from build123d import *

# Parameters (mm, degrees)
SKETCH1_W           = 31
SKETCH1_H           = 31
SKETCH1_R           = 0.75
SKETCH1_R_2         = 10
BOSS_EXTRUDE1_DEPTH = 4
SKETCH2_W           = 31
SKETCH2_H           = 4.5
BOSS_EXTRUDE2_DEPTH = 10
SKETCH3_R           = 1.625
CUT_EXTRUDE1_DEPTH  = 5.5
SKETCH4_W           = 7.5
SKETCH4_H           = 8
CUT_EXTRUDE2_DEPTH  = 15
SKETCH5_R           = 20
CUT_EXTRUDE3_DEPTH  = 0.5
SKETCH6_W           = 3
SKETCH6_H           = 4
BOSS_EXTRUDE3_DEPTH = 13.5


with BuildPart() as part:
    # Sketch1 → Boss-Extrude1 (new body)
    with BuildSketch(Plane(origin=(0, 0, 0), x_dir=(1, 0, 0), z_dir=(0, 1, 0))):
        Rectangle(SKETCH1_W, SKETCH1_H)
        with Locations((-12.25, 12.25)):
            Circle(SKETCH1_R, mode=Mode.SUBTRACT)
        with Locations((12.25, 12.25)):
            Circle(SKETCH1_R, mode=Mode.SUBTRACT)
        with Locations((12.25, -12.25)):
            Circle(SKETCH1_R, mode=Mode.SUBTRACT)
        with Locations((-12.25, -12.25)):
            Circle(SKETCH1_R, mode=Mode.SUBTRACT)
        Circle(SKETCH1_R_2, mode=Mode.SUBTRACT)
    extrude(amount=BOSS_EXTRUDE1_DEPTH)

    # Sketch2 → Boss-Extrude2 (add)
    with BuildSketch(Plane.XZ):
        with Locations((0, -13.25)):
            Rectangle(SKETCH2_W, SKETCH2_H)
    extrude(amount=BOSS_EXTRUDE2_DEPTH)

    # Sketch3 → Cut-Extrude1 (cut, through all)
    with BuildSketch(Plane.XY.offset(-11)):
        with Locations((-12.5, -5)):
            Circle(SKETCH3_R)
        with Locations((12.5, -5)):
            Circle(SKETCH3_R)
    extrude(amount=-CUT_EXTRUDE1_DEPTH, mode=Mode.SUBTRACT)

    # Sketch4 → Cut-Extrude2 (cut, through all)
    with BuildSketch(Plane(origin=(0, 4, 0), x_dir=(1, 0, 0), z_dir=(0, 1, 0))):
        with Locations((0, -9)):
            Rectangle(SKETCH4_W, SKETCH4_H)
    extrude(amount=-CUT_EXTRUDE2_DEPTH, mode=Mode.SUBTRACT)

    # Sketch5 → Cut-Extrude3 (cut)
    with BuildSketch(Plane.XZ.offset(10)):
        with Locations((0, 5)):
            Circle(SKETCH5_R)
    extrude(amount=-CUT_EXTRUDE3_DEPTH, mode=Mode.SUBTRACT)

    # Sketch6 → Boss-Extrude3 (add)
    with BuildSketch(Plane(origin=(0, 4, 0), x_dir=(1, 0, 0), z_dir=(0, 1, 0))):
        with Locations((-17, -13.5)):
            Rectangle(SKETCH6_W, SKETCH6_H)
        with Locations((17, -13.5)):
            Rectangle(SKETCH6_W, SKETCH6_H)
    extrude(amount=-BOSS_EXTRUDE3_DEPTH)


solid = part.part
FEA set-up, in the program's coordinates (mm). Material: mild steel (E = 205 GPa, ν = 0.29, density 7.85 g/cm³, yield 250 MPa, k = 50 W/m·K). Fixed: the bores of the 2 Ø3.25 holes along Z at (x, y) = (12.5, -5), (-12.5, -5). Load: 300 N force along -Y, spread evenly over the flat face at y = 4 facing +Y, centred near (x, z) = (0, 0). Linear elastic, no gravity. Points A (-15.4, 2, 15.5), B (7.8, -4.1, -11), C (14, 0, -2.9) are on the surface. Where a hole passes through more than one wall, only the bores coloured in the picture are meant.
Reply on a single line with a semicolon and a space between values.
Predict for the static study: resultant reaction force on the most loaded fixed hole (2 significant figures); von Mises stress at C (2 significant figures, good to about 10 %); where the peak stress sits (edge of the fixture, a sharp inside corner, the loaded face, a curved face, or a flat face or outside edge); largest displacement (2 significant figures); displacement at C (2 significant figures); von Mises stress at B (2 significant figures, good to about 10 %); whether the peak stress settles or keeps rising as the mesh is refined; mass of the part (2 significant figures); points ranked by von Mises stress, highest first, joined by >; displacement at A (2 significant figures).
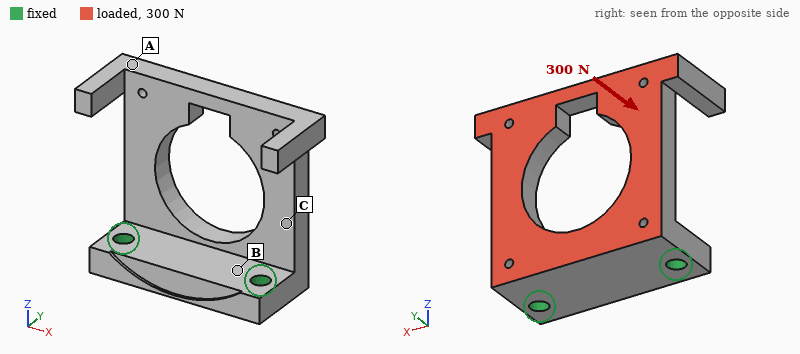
150 N; 56 MPa; a sharp inside corner; 77 µm; 15 µm; 26 MPa; keeps rising; 32 g; C > B > A; 69 µm
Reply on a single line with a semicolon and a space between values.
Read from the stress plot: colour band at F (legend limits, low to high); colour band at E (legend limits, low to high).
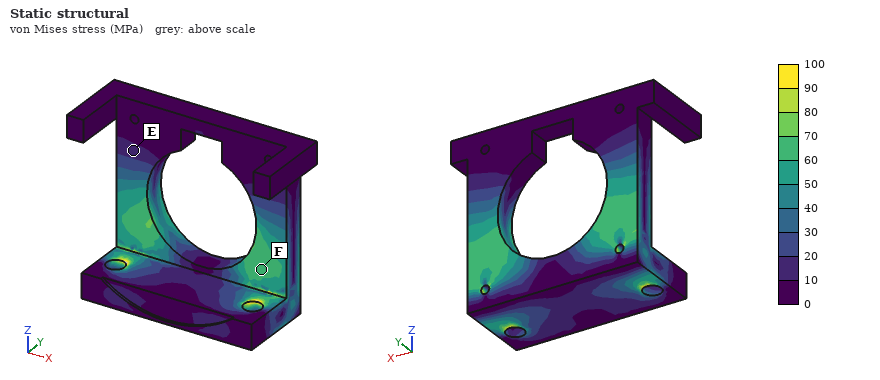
60 to 70 MPa; 10 to 20 MPa
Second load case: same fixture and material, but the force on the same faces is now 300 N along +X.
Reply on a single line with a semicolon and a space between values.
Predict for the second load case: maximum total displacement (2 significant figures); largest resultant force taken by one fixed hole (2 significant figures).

10 µm; 230 N
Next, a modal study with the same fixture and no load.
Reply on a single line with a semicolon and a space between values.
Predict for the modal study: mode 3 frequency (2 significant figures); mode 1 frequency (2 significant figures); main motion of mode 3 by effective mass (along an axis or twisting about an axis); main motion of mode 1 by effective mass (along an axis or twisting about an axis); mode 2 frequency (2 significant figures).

6500 Hz; 2400 Hz; along X; along Y; 4100 Hz
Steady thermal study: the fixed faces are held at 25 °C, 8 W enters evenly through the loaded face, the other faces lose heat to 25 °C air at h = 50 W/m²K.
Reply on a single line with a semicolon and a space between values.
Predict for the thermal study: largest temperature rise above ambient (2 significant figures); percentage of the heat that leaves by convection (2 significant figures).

31 K; 24 %
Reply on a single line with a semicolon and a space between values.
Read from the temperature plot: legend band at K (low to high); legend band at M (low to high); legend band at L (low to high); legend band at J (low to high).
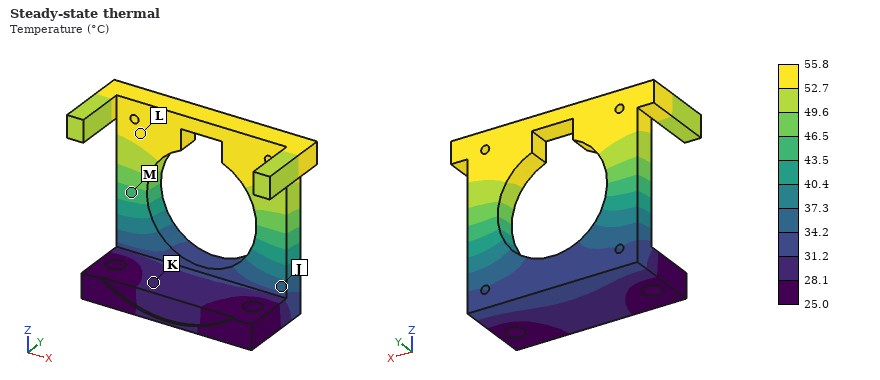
28.1 to 31.2 °C; 43.5 to 46.5 °C; 52.7 to 55.8 °C; 34.2 to 37.3 °C
